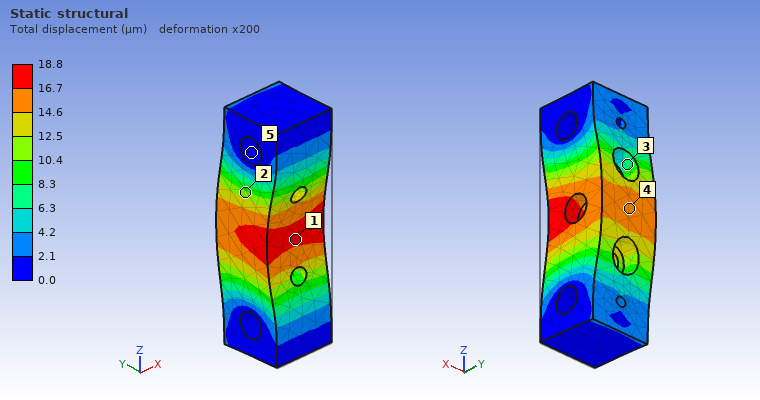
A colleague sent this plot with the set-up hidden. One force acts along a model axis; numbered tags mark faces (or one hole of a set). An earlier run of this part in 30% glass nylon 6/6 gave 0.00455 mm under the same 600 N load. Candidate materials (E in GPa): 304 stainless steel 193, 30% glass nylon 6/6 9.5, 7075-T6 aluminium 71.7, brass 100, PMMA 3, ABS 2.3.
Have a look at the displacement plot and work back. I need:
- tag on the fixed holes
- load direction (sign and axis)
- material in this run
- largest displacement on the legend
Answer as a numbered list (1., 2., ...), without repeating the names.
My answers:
1. 5
2. +Y
3. ABS
4. 18.8 µm
